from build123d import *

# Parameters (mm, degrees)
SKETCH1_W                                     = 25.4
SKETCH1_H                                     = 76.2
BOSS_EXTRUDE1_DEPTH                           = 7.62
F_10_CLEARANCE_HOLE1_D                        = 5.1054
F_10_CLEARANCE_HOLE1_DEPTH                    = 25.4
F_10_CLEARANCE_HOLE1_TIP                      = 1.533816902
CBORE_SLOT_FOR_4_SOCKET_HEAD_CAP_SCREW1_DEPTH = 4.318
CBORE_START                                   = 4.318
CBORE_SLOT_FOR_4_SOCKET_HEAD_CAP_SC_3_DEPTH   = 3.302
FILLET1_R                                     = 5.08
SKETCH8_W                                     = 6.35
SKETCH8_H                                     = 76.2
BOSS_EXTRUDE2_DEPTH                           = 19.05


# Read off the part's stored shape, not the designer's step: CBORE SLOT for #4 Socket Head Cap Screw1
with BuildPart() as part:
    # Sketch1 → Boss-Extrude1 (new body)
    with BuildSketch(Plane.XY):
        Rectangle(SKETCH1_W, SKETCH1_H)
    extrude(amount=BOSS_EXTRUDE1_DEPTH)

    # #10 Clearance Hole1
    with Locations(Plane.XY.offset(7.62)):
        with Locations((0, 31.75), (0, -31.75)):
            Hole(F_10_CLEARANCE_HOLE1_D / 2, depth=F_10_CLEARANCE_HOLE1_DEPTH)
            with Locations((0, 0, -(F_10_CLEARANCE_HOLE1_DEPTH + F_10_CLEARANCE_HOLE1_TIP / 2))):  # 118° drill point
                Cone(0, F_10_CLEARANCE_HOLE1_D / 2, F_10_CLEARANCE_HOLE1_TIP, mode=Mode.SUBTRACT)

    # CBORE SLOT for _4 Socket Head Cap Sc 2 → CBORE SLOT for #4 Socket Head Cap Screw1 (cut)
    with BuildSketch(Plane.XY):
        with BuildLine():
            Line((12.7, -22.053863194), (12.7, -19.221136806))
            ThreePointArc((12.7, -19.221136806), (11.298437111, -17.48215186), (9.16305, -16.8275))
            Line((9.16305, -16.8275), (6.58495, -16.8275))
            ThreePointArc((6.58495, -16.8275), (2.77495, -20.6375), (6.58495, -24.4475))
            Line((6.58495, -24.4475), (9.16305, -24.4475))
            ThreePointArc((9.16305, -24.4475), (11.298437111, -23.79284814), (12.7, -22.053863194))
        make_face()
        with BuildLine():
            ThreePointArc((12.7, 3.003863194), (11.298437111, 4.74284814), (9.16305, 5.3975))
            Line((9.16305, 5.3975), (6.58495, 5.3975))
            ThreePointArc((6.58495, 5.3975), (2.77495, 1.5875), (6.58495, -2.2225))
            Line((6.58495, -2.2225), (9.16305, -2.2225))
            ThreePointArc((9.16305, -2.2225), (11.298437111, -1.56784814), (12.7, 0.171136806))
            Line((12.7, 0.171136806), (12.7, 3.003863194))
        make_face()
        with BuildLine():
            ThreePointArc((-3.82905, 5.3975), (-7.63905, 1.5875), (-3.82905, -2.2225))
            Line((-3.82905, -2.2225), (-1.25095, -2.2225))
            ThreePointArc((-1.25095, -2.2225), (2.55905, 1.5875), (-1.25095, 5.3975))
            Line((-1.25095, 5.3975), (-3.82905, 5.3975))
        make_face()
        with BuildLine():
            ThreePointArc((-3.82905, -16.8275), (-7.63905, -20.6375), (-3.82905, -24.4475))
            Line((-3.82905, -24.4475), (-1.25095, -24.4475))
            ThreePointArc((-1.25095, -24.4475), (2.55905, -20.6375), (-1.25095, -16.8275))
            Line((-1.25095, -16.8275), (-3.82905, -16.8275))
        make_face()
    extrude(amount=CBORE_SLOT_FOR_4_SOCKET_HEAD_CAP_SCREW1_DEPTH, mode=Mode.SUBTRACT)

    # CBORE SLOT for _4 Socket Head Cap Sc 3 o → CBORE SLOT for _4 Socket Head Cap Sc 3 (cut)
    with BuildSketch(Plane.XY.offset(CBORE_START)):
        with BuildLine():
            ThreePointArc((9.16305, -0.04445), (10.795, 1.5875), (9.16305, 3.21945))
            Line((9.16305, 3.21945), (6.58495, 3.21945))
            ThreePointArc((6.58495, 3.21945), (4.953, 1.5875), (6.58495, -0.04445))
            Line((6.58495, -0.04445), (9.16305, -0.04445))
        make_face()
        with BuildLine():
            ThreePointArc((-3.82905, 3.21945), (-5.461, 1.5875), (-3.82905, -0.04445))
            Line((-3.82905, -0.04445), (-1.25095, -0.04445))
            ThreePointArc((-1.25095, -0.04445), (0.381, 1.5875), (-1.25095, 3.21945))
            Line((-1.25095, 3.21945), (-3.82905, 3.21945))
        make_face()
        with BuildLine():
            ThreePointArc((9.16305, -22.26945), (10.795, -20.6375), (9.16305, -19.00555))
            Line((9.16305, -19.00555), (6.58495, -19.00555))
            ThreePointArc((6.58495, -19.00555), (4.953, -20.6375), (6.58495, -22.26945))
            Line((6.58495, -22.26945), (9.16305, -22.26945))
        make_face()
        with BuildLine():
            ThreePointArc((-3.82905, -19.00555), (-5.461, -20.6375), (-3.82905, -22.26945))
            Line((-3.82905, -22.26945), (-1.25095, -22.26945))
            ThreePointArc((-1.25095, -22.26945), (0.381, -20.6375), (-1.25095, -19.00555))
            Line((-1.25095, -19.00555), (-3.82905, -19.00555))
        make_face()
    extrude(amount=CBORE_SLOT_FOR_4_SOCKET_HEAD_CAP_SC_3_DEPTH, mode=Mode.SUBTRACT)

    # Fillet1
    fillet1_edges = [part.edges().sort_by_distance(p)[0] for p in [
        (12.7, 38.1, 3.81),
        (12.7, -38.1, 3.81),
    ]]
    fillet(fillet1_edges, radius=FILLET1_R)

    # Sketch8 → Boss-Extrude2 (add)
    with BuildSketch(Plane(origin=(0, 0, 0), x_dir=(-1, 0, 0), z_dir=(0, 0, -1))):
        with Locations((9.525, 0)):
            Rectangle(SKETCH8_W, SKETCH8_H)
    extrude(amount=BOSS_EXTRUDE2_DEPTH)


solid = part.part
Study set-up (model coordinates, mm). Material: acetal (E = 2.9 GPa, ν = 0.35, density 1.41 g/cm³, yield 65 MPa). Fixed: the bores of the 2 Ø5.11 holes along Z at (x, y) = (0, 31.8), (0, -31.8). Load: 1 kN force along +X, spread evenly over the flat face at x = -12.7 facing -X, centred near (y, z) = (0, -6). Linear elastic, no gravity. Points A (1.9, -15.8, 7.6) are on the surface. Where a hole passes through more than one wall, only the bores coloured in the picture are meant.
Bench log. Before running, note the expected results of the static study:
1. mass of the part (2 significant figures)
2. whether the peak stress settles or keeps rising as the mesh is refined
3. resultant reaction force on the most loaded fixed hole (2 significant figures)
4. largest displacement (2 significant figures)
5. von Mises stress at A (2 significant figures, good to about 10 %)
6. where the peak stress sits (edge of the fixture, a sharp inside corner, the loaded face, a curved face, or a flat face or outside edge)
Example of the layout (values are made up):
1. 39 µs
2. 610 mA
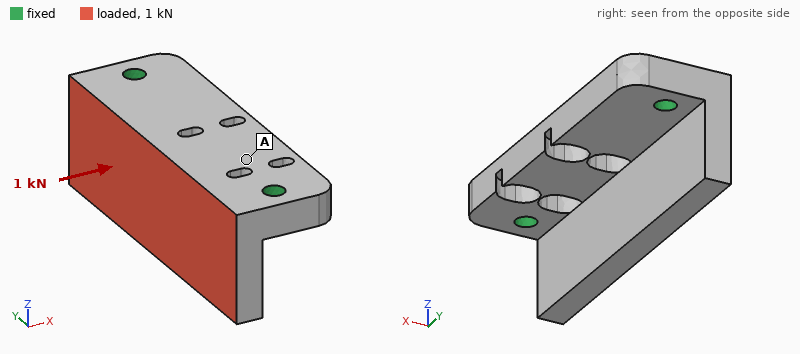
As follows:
1. 31 g
2. keeps rising
3. 520 N
4. 0.87 mm
5. 4.5 MPa
6. edge of the fixture
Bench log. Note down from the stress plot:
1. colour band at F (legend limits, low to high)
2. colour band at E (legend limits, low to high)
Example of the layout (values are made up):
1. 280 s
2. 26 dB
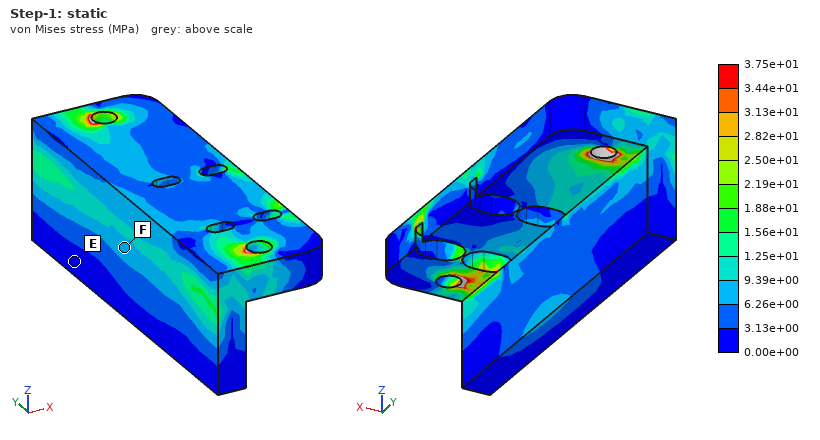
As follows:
1. 6.26e+00 to 9.39e+00 MPa
2. 0.00e+00 to 3.13e+00 MPa
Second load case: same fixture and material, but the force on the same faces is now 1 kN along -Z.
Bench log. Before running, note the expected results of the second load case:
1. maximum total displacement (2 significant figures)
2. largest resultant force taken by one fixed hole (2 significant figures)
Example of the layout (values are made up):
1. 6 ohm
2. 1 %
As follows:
1. 0.63 mm
2. 520 N
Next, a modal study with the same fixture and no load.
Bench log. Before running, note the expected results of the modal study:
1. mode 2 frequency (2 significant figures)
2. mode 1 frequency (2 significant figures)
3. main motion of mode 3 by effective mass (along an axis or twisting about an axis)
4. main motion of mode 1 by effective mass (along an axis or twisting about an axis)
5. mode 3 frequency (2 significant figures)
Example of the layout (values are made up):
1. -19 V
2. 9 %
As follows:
1. 2600 Hz
2. 1500 Hz
3. along Z
4. along X
5. 2700 Hz
